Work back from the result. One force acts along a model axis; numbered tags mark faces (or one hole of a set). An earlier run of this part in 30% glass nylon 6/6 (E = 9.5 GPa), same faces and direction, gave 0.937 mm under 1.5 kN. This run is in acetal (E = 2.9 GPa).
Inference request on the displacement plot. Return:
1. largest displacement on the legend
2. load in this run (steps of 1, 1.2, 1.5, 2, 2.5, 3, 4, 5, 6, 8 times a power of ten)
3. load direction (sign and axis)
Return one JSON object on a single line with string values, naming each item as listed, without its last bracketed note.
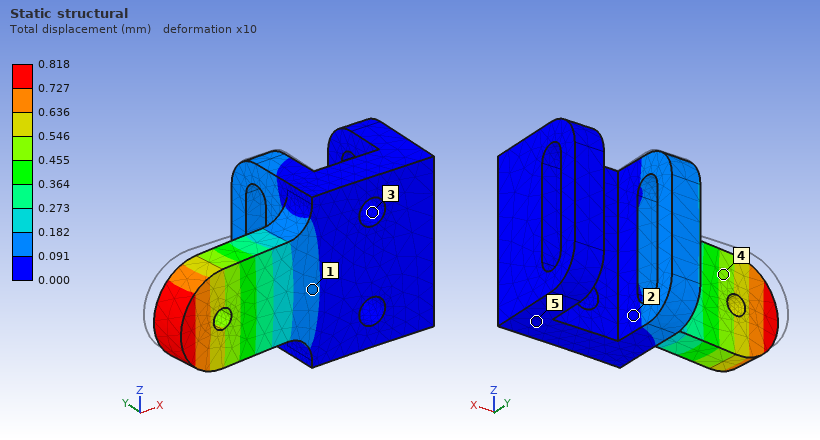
{"largest displacement on the legend": "0.818 mm", "load in this run": "400 N", "load direction": "-Y"}
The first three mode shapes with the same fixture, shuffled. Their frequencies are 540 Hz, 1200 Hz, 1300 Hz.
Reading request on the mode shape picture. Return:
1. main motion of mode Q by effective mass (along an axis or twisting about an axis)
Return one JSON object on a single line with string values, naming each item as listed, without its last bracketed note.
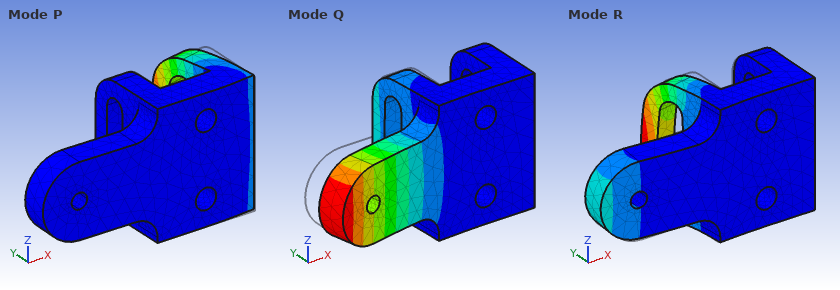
{"main motion of mode Q by effective mass": "along Y"}
